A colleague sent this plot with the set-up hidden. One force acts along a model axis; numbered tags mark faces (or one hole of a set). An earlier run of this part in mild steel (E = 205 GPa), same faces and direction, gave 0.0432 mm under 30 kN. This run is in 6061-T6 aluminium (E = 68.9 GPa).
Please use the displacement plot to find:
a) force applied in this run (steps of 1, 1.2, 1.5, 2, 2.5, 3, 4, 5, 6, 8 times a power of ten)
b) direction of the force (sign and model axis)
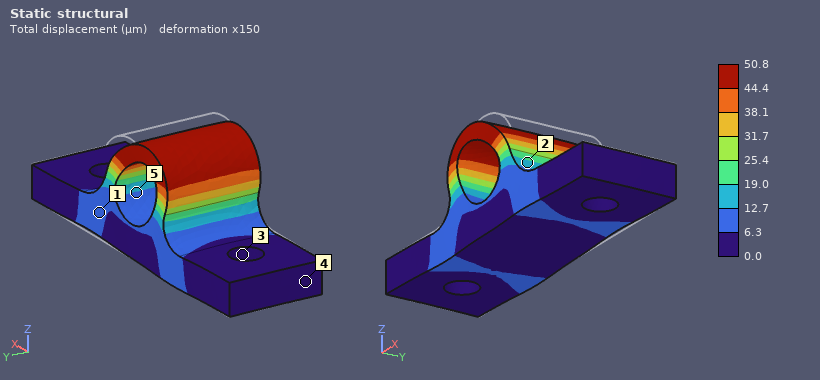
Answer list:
12 kN
-X
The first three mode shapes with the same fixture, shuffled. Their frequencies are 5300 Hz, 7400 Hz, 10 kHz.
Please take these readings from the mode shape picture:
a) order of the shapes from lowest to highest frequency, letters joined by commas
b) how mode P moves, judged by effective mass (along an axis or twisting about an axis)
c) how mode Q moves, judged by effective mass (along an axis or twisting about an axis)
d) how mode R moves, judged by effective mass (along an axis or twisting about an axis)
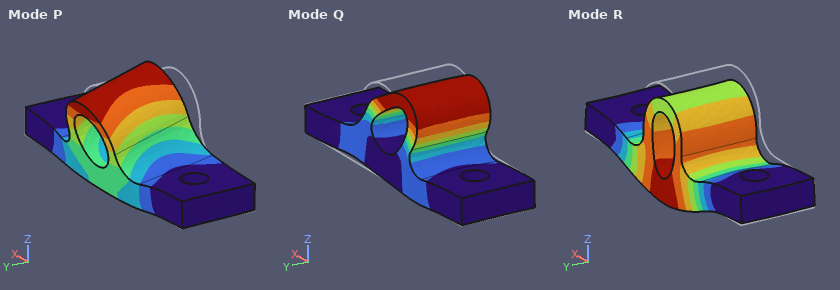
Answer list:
P, R, Q
along Y
along X
along Z
